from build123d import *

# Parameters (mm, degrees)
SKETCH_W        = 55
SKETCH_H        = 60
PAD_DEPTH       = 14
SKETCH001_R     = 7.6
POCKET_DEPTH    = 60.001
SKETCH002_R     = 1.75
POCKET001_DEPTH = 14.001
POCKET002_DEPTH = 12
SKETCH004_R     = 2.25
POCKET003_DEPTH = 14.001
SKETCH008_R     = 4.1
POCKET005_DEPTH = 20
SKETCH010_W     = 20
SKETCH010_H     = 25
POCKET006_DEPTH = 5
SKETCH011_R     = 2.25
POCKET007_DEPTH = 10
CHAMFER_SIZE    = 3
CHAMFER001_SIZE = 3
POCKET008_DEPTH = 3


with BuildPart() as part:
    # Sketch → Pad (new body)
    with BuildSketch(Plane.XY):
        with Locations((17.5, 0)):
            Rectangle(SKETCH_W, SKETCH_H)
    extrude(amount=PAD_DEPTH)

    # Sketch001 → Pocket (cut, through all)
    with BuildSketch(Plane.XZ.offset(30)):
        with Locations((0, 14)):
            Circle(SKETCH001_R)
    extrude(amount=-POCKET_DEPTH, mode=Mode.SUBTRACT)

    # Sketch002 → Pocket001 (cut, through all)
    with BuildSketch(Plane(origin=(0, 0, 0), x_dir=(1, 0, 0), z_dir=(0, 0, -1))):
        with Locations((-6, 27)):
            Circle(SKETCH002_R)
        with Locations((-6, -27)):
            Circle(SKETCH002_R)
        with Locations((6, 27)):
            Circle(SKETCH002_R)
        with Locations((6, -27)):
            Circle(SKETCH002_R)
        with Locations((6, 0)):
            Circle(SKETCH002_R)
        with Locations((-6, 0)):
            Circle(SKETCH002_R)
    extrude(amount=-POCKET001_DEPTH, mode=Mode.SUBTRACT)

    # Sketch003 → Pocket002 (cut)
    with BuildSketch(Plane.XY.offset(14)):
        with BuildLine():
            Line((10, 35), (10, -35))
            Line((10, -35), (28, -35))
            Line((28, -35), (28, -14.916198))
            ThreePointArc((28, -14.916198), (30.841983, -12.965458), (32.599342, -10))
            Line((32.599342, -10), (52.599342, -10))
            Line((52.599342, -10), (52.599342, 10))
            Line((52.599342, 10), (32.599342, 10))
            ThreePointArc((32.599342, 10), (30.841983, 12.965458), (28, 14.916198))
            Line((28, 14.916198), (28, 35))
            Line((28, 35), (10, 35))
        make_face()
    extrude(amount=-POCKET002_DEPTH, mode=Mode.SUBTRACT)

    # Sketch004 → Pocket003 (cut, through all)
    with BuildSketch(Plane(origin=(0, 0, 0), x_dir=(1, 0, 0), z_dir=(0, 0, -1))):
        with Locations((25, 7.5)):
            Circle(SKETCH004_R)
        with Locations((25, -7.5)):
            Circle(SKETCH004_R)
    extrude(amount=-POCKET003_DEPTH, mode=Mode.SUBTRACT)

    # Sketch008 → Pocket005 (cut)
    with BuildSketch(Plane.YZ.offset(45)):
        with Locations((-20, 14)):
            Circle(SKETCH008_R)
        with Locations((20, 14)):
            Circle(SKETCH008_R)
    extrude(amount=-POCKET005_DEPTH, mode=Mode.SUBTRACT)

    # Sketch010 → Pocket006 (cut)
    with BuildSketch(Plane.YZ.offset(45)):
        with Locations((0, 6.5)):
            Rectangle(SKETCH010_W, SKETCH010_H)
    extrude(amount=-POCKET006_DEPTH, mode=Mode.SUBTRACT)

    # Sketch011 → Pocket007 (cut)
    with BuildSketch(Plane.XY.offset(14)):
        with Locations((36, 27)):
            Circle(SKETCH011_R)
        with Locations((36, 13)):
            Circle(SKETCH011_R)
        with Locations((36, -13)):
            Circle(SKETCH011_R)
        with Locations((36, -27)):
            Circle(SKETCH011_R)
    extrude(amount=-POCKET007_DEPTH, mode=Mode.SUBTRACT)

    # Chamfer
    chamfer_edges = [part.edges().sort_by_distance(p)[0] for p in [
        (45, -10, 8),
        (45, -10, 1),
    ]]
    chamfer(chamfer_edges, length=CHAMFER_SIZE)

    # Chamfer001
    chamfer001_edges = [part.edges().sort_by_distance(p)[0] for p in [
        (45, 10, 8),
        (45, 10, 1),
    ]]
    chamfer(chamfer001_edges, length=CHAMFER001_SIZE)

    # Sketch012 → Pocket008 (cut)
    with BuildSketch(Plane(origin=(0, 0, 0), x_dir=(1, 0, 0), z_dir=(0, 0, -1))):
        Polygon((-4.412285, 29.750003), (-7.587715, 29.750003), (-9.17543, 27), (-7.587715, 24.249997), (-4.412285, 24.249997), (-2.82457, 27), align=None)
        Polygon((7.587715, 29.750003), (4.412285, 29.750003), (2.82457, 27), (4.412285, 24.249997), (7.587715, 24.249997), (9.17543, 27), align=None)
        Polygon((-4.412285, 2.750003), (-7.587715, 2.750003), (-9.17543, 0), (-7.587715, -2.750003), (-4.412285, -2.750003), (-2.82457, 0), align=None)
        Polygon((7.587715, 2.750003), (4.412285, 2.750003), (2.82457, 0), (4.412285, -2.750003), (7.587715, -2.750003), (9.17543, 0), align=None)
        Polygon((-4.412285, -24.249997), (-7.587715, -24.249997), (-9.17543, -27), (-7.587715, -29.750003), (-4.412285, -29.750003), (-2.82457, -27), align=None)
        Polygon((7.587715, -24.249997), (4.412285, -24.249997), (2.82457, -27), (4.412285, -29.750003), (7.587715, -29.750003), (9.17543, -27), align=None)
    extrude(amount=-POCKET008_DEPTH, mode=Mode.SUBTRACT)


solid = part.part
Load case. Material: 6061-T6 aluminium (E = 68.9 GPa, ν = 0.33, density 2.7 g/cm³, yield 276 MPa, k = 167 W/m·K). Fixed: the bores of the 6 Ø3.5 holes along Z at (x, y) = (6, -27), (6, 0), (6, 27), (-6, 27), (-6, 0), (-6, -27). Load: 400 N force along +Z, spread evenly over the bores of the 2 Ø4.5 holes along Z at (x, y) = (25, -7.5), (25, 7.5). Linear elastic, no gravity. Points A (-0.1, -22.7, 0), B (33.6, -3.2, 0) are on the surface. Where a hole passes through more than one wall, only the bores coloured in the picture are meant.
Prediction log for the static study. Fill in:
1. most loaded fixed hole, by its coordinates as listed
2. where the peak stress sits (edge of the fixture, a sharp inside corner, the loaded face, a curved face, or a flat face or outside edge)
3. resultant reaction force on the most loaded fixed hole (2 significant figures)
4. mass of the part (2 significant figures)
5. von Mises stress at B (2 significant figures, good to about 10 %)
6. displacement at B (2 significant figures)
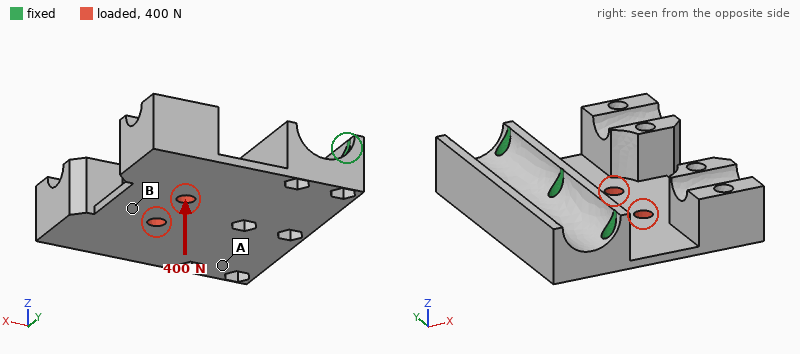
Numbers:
(6, 0)
a flat face or outside edge
560 N
56 g
30 MPa
0.39 mm
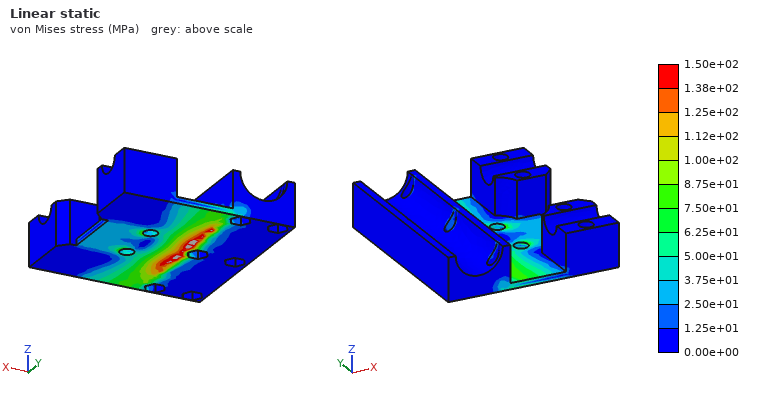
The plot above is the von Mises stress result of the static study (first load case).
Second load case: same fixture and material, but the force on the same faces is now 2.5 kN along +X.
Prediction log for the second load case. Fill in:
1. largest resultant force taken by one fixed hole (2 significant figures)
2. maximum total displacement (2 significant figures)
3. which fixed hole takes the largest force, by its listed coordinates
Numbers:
840 N
34 µm
(6, 0)
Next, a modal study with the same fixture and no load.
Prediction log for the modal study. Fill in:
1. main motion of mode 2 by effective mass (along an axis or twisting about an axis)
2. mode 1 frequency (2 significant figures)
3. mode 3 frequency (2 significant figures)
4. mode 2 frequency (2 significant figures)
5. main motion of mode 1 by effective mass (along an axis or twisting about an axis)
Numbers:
twisting about X
640 Hz
2500 Hz
1000 Hz
along Z
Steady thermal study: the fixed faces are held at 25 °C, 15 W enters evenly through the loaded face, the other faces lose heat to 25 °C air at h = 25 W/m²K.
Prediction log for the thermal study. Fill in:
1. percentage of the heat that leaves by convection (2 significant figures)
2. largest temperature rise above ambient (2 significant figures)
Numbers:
12 %
18 K
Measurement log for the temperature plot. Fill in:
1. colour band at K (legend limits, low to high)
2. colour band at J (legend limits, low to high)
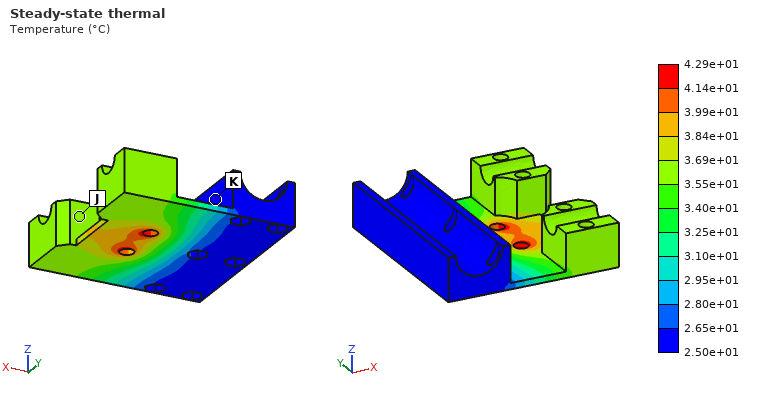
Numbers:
2.50e+01 to 2.65e+01 °C
3.55e+01 to 3.69e+01 °C
